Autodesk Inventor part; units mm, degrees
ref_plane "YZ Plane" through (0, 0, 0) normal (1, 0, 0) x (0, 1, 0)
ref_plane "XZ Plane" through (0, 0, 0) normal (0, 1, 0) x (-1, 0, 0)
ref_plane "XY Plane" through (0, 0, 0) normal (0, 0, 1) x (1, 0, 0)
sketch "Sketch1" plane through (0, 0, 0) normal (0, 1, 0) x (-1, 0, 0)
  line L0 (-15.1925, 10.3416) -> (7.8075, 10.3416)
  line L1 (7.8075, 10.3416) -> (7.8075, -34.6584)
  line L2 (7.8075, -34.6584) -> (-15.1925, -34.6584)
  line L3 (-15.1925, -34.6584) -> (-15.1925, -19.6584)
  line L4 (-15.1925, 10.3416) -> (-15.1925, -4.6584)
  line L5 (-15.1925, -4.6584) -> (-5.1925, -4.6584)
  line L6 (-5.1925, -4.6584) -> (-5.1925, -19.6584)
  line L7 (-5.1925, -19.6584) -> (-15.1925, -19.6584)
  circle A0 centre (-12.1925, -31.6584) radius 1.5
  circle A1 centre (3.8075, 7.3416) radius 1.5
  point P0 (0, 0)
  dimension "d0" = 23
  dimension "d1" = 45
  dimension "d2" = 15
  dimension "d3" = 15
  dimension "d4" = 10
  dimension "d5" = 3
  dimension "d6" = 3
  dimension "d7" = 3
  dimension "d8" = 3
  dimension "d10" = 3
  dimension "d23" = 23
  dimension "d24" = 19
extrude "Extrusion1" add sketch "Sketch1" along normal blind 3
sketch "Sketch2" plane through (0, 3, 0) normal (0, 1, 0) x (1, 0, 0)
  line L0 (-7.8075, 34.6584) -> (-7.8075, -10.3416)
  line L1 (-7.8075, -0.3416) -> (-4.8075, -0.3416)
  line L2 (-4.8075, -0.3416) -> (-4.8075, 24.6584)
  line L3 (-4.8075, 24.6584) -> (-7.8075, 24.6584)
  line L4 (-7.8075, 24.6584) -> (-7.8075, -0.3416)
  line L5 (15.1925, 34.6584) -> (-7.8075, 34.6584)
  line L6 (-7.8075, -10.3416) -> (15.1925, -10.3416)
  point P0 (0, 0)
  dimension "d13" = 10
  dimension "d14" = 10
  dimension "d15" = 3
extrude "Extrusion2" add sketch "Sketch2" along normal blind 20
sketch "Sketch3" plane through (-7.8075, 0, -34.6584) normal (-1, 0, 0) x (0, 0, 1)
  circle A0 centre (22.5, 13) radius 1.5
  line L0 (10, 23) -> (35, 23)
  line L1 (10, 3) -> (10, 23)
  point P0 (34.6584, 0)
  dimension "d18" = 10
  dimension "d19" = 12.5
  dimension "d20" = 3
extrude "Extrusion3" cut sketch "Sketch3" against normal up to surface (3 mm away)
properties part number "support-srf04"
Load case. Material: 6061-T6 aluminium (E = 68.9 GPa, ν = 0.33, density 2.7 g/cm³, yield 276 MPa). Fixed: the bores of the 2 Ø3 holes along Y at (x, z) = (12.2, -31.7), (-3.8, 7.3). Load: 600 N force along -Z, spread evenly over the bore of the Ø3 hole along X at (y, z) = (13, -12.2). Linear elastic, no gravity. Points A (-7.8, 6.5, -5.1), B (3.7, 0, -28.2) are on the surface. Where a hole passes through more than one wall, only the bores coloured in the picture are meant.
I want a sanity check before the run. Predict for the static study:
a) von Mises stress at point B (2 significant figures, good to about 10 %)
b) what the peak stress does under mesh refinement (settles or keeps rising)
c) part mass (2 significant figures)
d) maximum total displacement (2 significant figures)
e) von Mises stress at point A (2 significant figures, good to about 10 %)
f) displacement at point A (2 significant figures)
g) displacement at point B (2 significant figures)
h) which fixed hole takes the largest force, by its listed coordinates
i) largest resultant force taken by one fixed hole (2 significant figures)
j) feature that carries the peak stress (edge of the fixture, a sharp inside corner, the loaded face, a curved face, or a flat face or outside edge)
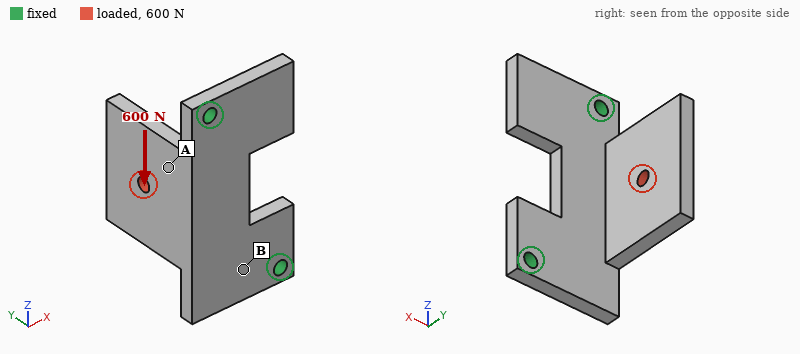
51 MPa
keeps rising
11 g
0.23 mm
21 MPa
0.051 mm
0.044 mm
(-3.8, 7.3)
550 N
edge of the fixture
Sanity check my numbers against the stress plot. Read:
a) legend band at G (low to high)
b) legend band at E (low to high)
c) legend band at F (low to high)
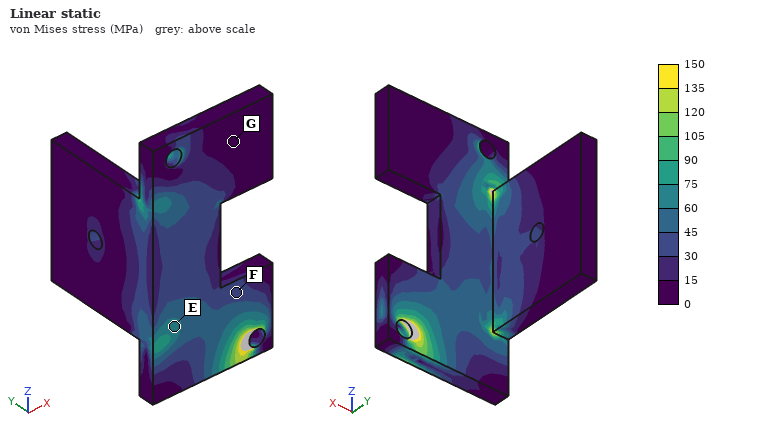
0 to 15 MPa
60 to 75 MPa
30 to 45 MPa
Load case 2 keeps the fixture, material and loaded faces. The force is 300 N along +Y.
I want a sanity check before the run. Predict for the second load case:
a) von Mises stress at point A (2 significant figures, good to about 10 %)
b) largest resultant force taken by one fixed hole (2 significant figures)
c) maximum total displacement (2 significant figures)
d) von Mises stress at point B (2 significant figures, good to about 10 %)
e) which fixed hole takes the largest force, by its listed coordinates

18 MPa
180 N
0.17 mm
36 MPa
(-3.8, 7.3)
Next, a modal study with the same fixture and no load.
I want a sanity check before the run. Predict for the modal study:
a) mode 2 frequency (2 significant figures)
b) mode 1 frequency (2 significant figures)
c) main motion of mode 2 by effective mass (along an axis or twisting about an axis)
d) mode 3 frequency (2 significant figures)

4700 Hz
2700 Hz
along Y
7100 Hz
